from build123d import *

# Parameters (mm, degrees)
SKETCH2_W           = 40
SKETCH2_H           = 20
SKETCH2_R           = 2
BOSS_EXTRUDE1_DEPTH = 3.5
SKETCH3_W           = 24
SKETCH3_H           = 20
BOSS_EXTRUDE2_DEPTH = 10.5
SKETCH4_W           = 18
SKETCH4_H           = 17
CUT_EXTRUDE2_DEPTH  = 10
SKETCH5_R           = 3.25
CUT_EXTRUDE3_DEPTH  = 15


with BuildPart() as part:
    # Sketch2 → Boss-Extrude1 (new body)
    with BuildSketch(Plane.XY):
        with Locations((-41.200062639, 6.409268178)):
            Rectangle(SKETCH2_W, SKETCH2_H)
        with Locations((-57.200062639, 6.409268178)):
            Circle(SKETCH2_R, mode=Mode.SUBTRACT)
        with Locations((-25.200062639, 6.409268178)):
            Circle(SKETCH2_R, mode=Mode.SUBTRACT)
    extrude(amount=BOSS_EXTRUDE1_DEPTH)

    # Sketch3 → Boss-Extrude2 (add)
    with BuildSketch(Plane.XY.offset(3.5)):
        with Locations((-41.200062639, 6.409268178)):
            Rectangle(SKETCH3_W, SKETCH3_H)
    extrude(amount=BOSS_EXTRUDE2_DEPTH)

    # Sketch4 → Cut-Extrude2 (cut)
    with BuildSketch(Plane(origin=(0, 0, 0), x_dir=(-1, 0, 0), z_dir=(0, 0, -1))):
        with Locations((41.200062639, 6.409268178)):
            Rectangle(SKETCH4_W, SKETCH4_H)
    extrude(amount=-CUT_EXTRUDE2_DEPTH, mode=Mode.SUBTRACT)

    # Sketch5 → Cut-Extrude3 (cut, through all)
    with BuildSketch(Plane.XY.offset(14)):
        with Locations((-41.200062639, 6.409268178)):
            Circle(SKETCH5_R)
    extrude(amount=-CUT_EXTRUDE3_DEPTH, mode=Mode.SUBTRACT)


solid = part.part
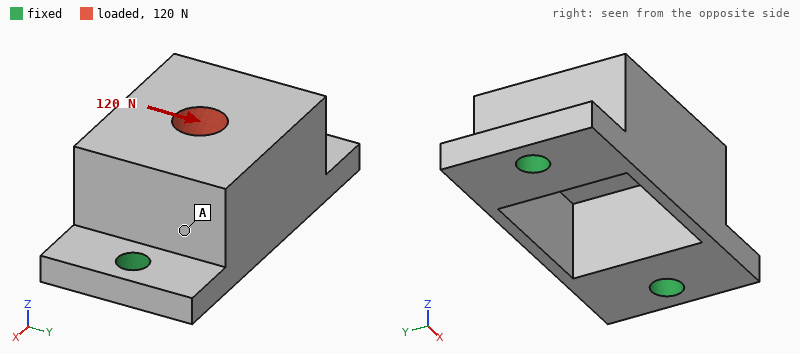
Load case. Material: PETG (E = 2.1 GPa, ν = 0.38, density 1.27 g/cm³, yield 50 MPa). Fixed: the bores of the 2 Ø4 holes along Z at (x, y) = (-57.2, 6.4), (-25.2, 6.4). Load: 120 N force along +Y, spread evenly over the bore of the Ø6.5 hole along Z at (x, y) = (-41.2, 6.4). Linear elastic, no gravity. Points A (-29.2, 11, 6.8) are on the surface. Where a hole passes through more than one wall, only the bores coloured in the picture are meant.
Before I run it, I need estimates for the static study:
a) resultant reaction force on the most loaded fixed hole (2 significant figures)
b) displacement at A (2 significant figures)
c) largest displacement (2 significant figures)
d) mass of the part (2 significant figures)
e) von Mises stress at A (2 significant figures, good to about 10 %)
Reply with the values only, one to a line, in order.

60 N
0.098 mm
0.23 mm
5.8 g
3.0 MPa
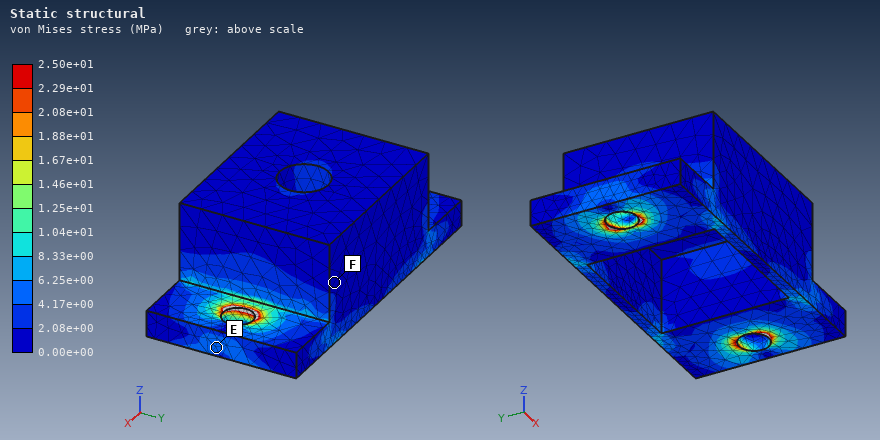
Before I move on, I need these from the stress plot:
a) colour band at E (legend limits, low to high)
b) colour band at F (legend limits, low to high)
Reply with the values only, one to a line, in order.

4.17e+00 to 6.25e+00 MPa
0.00e+00 to 2.08e+00 MPa
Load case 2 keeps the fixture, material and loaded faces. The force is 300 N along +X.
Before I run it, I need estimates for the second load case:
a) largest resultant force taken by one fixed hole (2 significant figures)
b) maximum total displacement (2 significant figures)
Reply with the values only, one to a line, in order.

180 N
0.11 mm
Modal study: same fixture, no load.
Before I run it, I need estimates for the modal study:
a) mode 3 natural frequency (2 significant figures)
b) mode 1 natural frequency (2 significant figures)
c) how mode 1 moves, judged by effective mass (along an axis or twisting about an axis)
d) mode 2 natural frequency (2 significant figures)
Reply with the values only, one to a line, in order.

5300 Hz
2100 Hz
along Y
5300 Hz
